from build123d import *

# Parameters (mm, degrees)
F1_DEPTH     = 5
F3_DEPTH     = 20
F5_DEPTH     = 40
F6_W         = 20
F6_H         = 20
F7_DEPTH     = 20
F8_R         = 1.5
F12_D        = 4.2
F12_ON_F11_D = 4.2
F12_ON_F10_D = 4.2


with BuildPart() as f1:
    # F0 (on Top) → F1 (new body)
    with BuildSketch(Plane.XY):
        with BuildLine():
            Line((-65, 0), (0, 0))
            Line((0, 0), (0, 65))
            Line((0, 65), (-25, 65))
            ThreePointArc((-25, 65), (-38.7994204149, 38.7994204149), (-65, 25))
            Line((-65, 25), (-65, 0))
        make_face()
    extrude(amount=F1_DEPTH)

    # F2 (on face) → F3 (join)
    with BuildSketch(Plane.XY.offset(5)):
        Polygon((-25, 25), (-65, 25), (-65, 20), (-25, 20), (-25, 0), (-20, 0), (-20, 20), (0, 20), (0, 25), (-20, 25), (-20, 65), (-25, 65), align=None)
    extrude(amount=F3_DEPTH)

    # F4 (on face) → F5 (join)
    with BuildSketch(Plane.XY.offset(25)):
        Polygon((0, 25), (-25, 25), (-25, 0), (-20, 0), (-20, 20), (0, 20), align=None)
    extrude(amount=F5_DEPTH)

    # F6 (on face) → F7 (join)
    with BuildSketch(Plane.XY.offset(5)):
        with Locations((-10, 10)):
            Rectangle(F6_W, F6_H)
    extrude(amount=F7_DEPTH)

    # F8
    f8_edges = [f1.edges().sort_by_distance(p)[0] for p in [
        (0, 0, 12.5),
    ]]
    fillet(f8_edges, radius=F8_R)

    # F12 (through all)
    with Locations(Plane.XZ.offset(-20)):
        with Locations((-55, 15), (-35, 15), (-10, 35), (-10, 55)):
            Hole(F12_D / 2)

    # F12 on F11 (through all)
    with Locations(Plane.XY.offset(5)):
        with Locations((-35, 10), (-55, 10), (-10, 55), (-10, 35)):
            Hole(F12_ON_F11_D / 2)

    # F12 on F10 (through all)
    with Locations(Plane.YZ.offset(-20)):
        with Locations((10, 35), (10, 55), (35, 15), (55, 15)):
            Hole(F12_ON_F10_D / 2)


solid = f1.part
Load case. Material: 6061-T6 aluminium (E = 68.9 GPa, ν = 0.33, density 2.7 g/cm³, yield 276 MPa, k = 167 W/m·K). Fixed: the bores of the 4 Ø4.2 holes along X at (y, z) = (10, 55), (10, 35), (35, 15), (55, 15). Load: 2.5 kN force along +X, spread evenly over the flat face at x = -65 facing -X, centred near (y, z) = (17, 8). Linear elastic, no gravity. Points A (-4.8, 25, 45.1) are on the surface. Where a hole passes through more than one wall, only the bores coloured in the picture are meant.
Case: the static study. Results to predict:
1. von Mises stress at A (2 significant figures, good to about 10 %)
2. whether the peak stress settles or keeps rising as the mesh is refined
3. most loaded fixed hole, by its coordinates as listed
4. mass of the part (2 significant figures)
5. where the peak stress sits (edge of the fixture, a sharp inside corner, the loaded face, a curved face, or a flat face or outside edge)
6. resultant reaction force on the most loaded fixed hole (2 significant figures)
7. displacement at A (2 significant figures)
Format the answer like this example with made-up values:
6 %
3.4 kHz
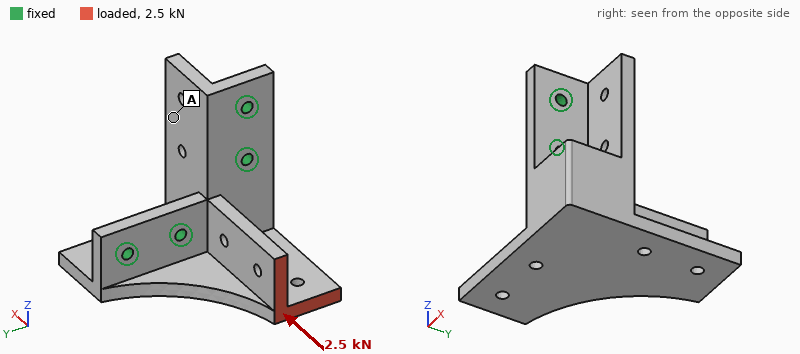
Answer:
12 MPa
keeps rising
(35, 15)
120 g
edge of the fixture
2.1 kN
0.047 mm
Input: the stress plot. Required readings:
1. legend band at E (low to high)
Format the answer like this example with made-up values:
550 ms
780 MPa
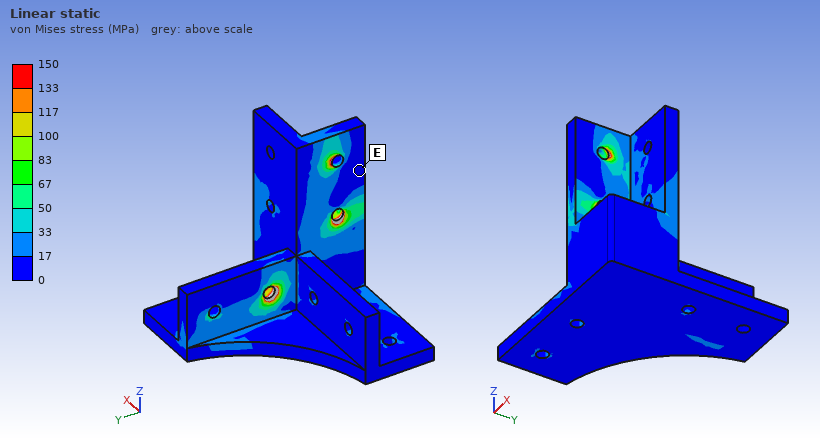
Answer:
0 to 17 MPa
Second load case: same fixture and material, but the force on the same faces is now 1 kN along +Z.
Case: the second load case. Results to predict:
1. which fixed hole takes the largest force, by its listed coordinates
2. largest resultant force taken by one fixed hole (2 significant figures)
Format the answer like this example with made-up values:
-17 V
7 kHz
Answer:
(35, 15)
1.2 kN
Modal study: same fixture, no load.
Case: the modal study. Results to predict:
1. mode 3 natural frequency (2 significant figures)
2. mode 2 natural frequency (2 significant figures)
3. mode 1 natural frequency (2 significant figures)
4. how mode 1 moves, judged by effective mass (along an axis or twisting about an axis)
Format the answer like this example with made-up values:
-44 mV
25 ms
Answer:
5700 Hz
5200 Hz
2700 Hz
along X
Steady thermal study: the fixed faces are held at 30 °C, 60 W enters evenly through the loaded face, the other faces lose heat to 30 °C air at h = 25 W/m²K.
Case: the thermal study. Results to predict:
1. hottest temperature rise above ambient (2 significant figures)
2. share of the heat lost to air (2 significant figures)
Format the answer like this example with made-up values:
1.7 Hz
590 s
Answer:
73 K
12 %
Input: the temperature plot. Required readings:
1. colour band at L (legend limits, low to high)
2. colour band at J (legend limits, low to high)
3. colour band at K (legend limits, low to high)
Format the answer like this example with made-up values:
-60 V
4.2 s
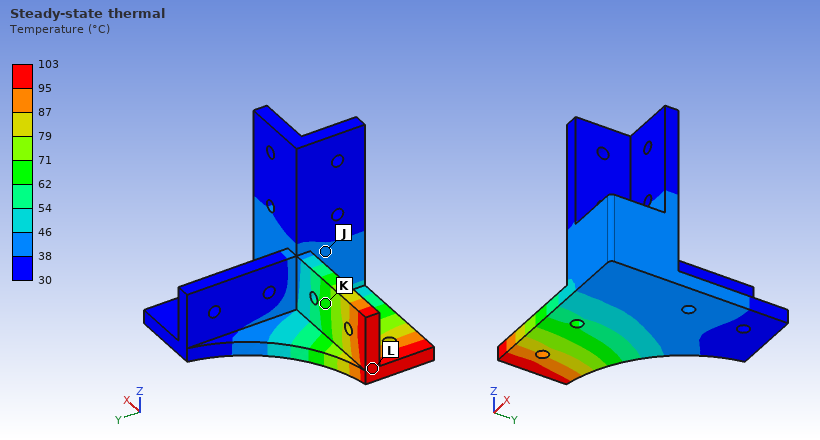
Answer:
95 to 103 °C
38 to 46 °C
62 to 71 °C
